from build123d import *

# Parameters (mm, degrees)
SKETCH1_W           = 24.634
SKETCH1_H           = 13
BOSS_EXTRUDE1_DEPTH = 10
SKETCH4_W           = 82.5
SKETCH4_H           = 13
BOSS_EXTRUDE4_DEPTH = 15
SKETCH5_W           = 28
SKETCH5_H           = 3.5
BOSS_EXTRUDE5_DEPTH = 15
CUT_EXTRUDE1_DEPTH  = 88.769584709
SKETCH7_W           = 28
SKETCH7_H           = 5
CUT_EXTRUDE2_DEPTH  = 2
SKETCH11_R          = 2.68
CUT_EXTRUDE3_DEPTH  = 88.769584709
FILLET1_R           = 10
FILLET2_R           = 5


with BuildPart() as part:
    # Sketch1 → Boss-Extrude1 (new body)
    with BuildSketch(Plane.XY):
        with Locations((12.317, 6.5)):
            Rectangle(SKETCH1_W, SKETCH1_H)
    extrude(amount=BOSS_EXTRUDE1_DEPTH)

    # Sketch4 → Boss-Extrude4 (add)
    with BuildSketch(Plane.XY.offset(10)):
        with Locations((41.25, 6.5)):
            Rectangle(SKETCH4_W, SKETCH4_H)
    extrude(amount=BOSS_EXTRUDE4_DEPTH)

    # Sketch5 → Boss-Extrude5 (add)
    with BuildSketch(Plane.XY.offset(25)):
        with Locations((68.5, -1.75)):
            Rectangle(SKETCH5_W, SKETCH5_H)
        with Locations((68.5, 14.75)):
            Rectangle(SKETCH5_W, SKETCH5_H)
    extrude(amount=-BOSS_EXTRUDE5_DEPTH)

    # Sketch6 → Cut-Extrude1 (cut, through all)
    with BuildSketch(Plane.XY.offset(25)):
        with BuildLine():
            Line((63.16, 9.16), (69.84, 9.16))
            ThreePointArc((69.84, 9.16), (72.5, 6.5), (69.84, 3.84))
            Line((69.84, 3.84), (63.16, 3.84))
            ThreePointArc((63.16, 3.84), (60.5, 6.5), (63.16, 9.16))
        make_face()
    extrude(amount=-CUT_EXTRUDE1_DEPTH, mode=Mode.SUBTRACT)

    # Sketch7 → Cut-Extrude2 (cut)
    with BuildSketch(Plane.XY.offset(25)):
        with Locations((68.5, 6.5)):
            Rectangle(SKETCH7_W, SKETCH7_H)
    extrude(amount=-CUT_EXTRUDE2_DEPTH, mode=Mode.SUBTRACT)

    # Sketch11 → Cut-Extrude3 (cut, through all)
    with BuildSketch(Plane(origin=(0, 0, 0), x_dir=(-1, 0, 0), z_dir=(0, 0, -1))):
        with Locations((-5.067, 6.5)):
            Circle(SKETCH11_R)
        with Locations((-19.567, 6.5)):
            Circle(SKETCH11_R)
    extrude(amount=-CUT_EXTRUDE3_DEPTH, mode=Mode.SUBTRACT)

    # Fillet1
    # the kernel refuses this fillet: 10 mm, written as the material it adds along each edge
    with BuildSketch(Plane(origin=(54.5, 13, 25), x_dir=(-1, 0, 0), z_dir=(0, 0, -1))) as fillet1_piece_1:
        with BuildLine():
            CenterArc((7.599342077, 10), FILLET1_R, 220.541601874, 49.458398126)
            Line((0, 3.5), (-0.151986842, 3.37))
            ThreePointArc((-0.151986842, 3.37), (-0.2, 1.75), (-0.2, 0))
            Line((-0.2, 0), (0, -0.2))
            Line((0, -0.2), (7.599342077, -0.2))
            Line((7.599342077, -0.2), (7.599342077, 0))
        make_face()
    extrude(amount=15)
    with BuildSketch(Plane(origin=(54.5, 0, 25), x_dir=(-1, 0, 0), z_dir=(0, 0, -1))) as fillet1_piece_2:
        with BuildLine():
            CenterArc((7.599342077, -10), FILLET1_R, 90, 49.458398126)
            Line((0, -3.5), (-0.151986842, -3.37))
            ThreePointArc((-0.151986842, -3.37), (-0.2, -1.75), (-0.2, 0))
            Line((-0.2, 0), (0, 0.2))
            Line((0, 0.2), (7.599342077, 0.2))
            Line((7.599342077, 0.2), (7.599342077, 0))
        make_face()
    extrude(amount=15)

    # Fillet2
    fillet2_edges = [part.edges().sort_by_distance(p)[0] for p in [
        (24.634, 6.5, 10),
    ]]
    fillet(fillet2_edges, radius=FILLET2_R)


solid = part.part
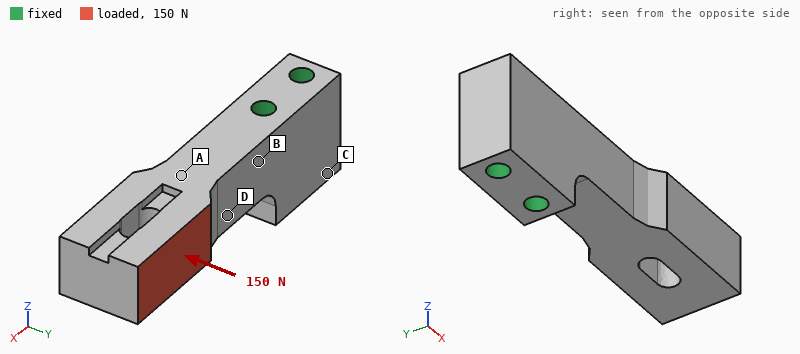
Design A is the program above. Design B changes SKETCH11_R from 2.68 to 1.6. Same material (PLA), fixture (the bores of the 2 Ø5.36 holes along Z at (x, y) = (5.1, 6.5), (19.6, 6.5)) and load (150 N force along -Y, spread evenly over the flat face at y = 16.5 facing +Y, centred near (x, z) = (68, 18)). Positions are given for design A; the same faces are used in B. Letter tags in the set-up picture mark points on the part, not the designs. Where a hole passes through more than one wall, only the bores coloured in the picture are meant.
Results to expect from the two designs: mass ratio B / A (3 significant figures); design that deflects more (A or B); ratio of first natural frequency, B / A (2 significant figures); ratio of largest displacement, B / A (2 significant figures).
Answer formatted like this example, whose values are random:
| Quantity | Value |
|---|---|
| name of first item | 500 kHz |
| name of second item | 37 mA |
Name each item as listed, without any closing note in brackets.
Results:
| Quantity | Value |
|---|---|
| mass ratio B / A | 1.04 |
| design that deflects more | B |
| ratio of first natural frequency, B / A | 0.94 |
| ratio of largest displacement, B / A | 1.1 |
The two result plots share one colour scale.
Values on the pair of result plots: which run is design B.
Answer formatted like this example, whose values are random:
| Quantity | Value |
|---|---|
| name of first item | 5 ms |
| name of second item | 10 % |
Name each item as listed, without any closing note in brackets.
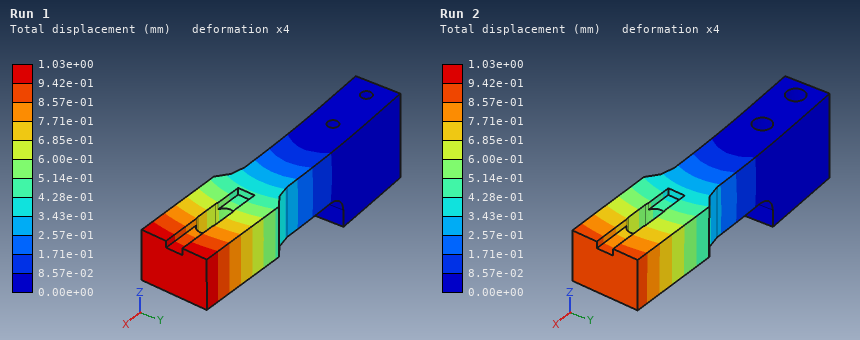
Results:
| Quantity | Value |
|---|---|
| which run is design B | Run 1 |
